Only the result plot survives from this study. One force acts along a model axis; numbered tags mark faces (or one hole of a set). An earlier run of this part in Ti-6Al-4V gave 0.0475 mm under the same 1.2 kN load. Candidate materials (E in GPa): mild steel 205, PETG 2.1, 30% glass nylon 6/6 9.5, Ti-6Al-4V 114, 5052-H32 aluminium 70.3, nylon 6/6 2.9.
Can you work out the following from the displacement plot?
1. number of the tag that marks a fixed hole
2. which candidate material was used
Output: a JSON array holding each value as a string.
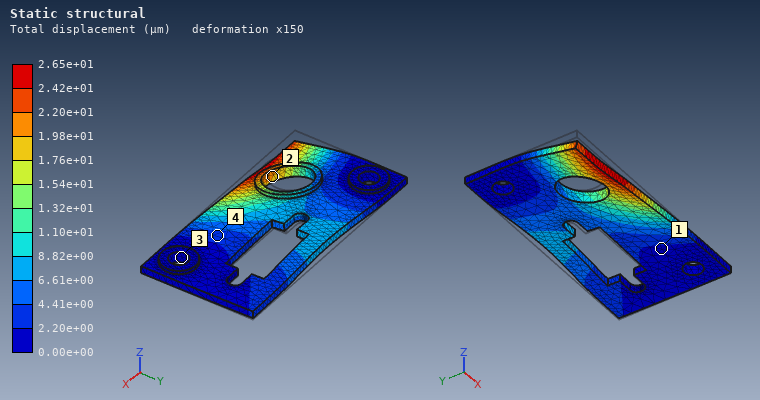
["3", "mild steel"]
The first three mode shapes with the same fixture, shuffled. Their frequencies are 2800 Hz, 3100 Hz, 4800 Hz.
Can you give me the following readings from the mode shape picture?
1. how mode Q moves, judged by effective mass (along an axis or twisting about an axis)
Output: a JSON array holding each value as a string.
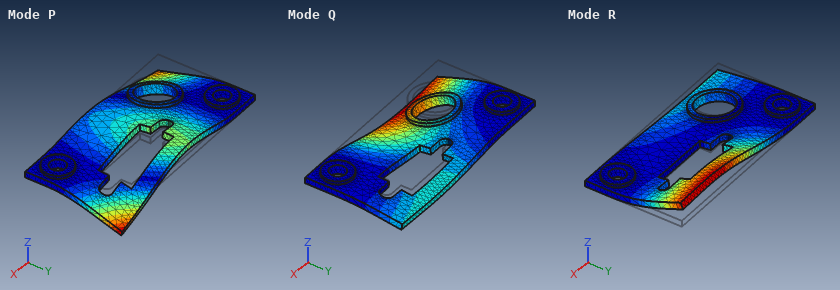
["along Z"]
